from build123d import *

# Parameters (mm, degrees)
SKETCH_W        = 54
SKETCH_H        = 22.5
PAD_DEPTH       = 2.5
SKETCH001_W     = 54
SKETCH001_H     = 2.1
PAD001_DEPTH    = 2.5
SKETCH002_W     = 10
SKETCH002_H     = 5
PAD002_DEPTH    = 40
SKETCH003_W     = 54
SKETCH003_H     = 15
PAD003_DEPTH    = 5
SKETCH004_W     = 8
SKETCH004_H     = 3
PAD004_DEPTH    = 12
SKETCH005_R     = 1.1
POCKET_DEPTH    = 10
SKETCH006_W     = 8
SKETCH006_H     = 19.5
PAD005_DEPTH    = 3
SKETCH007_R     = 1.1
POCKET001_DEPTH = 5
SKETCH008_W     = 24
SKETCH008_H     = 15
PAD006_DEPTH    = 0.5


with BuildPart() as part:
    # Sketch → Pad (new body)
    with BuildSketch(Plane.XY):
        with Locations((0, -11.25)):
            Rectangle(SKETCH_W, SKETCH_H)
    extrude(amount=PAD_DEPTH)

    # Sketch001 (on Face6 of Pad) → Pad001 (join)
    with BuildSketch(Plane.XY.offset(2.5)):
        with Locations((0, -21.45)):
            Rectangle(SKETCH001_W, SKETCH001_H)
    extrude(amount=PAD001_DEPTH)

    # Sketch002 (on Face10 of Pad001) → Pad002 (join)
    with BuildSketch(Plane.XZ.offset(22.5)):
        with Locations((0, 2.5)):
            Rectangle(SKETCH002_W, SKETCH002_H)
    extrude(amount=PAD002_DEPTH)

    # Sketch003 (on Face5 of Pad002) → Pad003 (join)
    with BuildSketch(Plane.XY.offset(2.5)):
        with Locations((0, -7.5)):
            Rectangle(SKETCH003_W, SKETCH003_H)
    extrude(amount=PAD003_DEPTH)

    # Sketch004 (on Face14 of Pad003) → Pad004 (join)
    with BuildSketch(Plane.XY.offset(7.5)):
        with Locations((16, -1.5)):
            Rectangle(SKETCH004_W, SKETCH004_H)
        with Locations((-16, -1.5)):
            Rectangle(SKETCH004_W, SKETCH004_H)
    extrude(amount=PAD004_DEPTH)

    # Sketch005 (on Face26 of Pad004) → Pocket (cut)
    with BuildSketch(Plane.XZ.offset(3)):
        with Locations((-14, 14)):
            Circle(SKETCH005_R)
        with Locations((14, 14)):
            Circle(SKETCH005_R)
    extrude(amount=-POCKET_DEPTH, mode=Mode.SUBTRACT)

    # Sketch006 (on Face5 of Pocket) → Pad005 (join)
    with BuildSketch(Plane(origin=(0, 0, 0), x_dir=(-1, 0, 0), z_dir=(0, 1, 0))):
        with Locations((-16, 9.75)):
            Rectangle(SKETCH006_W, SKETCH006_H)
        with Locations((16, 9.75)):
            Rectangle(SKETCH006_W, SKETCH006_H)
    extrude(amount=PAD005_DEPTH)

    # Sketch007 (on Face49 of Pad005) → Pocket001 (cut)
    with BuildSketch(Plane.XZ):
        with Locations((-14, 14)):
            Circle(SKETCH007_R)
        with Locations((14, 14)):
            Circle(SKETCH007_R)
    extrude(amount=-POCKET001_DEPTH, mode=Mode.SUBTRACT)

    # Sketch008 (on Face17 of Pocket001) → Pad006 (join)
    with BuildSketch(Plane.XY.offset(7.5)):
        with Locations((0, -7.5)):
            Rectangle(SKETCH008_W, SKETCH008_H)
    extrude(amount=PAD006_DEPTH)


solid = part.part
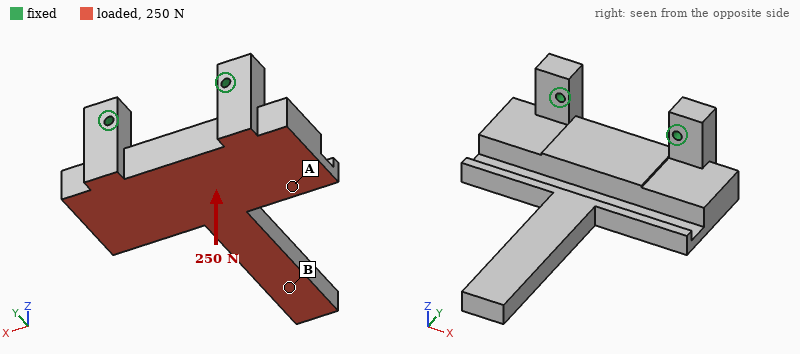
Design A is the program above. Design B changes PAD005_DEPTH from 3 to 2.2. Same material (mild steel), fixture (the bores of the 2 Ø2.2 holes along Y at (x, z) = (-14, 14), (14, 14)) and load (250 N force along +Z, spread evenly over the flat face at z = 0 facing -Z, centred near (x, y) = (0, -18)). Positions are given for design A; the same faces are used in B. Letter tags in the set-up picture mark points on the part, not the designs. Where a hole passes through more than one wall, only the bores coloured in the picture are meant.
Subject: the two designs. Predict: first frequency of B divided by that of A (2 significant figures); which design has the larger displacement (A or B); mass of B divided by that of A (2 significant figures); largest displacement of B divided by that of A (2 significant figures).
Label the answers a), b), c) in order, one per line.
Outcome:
a) 0.95
b) B
c) 0.98
d) 1.1
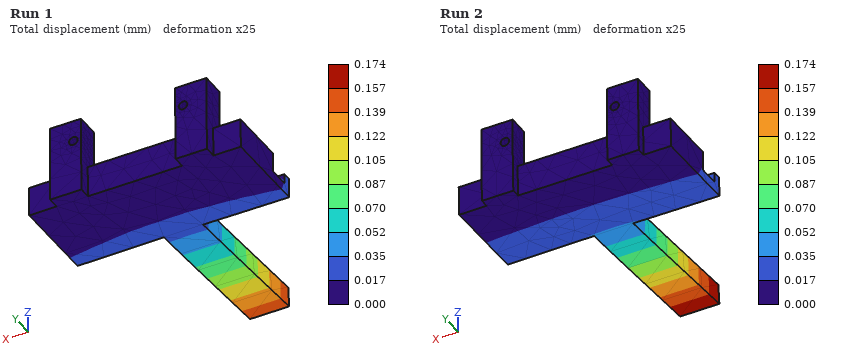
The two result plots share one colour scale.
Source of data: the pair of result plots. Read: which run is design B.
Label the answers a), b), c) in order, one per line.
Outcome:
a) Run 2
